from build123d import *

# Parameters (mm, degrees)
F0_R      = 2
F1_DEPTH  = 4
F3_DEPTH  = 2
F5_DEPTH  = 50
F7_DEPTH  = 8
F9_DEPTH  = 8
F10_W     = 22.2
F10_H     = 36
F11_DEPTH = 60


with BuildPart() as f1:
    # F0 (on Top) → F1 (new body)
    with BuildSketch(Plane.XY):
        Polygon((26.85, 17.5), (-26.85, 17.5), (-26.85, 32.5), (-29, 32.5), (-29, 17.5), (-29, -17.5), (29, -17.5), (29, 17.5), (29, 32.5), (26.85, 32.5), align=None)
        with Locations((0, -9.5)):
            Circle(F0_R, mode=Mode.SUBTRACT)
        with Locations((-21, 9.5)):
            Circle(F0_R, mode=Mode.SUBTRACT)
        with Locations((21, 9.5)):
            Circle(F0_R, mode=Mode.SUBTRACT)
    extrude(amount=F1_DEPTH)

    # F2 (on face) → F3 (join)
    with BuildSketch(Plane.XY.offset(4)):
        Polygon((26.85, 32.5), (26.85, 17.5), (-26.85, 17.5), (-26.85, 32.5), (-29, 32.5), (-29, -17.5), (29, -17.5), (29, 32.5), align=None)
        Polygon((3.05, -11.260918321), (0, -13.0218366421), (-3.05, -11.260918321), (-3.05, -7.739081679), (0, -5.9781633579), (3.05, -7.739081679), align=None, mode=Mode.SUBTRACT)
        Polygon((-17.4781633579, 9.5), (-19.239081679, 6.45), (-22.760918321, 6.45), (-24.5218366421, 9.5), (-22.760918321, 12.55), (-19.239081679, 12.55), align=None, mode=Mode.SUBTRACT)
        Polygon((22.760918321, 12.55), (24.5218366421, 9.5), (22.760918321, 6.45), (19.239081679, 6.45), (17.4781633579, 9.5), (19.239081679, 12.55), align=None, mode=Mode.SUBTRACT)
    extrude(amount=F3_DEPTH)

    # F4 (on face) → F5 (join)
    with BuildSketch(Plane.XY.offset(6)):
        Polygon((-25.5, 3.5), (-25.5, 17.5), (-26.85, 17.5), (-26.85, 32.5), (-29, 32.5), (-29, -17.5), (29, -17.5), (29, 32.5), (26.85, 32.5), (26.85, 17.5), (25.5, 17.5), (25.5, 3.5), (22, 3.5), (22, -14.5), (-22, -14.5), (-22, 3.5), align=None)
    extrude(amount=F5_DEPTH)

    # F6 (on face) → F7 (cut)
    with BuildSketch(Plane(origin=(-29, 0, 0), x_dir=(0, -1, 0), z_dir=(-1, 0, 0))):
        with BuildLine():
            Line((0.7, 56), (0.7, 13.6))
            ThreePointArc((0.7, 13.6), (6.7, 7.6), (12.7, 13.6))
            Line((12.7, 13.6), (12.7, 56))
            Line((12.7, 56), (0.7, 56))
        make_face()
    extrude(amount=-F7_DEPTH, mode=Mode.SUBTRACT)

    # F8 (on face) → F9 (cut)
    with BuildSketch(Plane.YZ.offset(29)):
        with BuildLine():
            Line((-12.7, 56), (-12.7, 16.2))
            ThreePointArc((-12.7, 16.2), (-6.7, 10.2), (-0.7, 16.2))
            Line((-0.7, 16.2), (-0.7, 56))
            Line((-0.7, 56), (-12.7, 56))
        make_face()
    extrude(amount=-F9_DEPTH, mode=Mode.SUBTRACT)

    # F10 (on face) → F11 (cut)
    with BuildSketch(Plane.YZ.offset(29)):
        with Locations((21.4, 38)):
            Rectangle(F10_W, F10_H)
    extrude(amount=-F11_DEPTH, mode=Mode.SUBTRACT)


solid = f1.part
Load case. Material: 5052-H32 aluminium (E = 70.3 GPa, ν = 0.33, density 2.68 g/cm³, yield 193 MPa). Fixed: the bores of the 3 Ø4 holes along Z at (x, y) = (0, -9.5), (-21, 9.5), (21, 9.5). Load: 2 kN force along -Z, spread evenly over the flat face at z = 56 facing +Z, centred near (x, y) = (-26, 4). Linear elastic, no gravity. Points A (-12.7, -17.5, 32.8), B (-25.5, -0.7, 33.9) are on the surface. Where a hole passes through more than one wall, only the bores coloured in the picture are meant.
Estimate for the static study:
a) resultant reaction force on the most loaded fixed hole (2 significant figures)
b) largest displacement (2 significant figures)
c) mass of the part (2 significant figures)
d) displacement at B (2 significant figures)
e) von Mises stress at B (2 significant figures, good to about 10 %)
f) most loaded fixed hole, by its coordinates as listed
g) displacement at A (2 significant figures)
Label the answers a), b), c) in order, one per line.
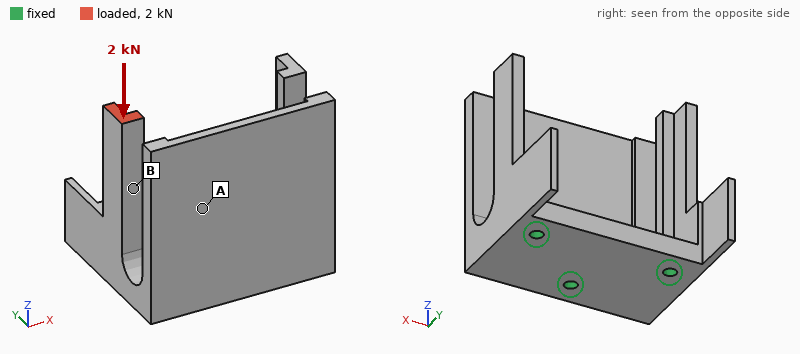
a) 1.9 kN
b) 0.15 mm
c) 80 g
d) 0.090 mm
e) 38 MPa
f) (-21, 9.5)
g) 0.032 mm
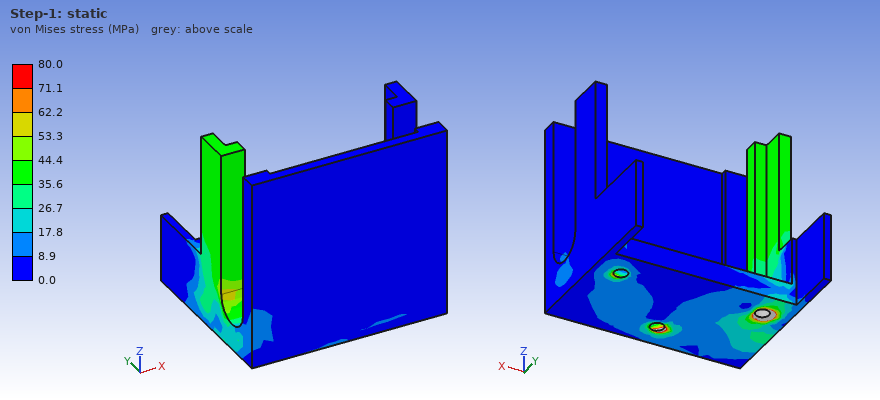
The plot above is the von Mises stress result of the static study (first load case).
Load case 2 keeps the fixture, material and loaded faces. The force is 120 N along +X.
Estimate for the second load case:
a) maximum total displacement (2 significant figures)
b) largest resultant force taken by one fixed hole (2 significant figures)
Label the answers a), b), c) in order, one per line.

a) 0.51 mm
b) 110 N
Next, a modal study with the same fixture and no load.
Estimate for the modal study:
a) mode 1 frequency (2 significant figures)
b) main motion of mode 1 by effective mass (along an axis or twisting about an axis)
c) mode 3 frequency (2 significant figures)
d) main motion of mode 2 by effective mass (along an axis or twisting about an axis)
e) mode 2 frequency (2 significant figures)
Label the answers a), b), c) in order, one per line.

a) 1300 Hz
b) along Y
c) 1900 Hz
d) along X
e) 1700 Hz
